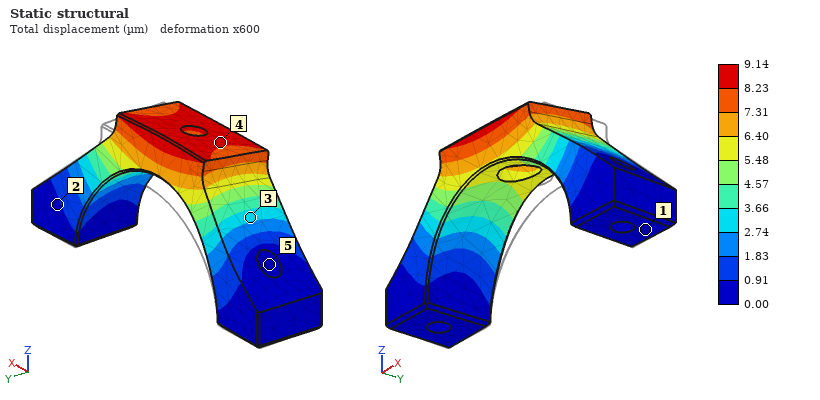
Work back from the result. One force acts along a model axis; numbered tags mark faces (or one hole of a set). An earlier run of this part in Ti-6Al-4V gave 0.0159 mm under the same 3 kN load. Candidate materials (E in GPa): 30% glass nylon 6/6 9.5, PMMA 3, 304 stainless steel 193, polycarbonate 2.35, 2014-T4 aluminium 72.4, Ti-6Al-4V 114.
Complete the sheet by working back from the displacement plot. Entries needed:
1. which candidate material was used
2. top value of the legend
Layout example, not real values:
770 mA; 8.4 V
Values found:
304 stainless steel; 9.14 µm
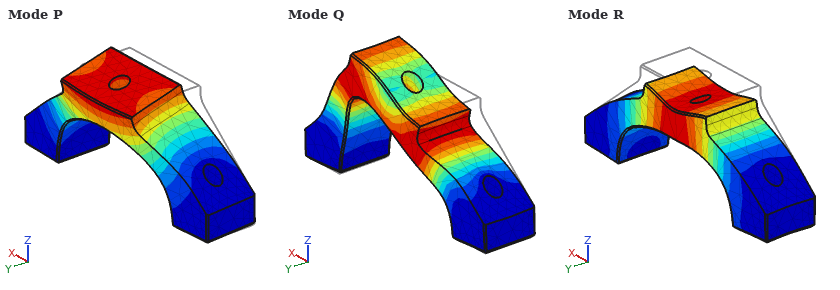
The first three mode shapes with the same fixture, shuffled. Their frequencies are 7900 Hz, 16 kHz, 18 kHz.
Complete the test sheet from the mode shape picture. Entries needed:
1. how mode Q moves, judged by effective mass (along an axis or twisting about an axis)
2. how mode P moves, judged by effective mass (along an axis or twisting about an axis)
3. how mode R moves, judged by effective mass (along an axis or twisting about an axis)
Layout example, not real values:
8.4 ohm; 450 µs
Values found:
along X; along Y; along Z
